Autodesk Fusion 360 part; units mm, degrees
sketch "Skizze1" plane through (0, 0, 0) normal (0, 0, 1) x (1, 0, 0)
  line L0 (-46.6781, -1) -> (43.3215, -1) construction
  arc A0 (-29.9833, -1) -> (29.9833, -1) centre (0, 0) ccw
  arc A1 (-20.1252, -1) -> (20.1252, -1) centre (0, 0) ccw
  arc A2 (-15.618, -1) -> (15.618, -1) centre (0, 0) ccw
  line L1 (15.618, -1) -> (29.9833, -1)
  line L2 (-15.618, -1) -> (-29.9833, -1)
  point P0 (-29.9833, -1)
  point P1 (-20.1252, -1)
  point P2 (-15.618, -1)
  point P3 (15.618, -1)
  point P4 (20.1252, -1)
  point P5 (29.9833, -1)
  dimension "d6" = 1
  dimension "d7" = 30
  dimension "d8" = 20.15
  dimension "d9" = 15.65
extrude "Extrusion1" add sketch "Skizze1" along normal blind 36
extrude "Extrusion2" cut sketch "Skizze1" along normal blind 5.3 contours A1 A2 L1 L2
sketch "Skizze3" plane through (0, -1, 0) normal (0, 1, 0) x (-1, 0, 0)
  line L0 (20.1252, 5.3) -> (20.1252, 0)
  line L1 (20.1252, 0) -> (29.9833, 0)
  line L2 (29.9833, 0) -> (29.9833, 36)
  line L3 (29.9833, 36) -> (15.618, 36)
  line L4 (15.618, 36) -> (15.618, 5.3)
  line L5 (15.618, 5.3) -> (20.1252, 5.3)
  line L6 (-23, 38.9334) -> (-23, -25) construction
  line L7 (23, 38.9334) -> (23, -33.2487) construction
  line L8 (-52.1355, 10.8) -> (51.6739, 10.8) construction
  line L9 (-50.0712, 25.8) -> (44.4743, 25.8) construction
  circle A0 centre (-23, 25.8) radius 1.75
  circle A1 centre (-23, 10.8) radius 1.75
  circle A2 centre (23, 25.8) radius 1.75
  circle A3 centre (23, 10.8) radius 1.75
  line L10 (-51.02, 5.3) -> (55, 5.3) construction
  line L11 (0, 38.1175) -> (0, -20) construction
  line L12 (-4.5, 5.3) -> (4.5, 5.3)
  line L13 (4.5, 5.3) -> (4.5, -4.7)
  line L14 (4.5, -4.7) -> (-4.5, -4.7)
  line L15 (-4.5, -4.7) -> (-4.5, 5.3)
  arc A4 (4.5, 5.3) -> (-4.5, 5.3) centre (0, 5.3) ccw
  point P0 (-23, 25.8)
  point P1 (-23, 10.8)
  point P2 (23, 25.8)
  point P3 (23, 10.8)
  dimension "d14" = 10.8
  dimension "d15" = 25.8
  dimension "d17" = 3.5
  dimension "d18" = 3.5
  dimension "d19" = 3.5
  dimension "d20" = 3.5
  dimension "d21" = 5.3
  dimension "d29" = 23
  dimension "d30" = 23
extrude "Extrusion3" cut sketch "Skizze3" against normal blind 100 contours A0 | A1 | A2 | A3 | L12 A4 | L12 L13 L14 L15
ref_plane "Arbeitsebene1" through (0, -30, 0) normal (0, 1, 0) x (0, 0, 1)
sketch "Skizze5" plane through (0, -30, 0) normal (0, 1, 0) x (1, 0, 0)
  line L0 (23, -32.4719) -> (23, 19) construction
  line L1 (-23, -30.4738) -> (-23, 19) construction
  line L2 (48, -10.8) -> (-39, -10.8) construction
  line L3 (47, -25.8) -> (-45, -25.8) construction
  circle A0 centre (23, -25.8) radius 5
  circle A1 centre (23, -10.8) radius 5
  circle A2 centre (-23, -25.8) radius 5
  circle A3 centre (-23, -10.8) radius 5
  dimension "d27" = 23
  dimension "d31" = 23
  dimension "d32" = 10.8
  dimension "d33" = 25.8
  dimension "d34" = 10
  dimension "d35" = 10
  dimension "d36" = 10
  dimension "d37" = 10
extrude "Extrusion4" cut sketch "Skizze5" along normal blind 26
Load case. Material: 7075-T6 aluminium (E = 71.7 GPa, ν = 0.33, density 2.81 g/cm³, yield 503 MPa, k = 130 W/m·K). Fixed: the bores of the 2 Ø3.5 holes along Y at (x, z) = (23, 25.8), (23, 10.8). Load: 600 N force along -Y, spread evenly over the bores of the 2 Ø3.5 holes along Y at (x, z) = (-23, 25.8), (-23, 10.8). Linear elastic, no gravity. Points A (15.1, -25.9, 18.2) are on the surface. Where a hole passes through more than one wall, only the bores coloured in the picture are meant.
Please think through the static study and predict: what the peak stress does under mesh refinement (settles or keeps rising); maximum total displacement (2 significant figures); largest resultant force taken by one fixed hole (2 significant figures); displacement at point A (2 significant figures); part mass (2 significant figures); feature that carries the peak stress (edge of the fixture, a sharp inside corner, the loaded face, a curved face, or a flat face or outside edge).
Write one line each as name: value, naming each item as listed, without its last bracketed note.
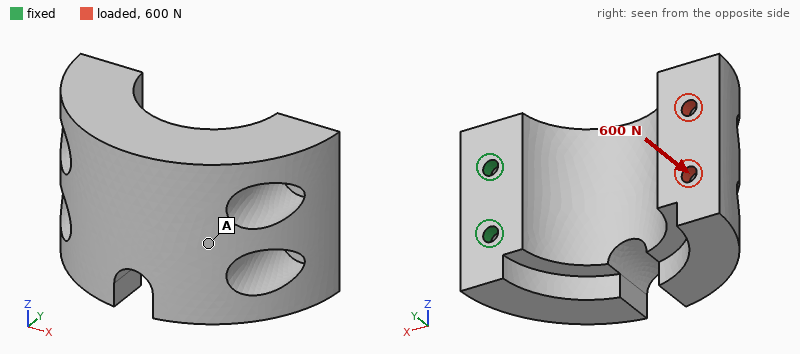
what the peak stress does under mesh refinement: keeps rising
maximum total displacement: 0.45 mm
largest resultant force taken by one fixed hole: 360 N
displacement at point A: 0.19 mm
part mass: 82 g
feature that carries the peak stress: edge of the fixture
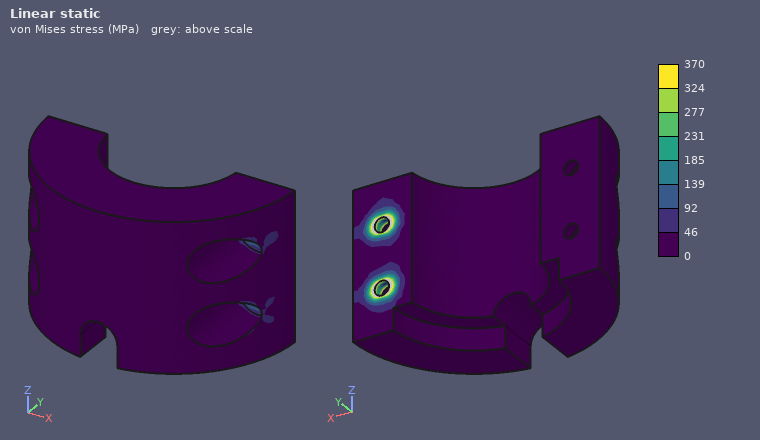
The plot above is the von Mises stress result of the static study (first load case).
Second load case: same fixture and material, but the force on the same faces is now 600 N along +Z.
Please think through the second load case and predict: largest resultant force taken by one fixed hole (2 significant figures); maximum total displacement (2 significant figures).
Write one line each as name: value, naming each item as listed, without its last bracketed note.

largest resultant force taken by one fixed hole: 1.5 kN
maximum total displacement: 0.13 mm
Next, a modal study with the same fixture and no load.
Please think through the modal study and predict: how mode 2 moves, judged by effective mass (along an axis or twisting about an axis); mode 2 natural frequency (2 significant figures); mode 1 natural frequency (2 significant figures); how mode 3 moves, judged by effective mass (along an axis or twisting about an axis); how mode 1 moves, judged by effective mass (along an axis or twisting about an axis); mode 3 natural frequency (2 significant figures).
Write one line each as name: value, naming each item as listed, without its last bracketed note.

how mode 2 moves, judged by effective mass: along Z
mode 2 natural frequency: 2500 Hz
mode 1 natural frequency: 1000 Hz
how mode 3 moves, judged by effective mass: along Z
how mode 1 moves, judged by effective mass: along Y
mode 3 natural frequency: 4300 Hz
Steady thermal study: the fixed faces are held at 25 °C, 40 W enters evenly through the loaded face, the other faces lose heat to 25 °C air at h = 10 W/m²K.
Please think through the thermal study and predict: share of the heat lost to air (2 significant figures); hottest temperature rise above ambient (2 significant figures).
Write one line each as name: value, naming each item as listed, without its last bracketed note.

share of the heat lost to air: 8.2 %
hottest temperature rise above ambient: 71 K
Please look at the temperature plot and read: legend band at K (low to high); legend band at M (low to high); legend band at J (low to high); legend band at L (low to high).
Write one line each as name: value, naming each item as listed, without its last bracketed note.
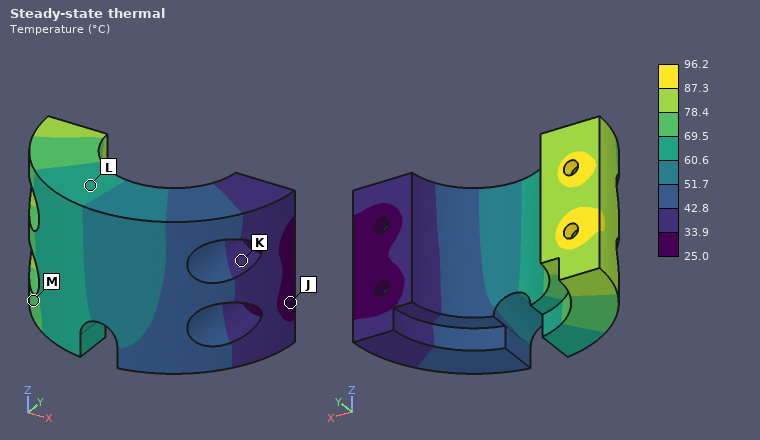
legend band at K: 33.9 to 42.8 °C
legend band at M: 69.5 to 78.4 °C
legend band at J: 25.0 to 33.9 °C
legend band at L: 60.6 to 69.5 °C
